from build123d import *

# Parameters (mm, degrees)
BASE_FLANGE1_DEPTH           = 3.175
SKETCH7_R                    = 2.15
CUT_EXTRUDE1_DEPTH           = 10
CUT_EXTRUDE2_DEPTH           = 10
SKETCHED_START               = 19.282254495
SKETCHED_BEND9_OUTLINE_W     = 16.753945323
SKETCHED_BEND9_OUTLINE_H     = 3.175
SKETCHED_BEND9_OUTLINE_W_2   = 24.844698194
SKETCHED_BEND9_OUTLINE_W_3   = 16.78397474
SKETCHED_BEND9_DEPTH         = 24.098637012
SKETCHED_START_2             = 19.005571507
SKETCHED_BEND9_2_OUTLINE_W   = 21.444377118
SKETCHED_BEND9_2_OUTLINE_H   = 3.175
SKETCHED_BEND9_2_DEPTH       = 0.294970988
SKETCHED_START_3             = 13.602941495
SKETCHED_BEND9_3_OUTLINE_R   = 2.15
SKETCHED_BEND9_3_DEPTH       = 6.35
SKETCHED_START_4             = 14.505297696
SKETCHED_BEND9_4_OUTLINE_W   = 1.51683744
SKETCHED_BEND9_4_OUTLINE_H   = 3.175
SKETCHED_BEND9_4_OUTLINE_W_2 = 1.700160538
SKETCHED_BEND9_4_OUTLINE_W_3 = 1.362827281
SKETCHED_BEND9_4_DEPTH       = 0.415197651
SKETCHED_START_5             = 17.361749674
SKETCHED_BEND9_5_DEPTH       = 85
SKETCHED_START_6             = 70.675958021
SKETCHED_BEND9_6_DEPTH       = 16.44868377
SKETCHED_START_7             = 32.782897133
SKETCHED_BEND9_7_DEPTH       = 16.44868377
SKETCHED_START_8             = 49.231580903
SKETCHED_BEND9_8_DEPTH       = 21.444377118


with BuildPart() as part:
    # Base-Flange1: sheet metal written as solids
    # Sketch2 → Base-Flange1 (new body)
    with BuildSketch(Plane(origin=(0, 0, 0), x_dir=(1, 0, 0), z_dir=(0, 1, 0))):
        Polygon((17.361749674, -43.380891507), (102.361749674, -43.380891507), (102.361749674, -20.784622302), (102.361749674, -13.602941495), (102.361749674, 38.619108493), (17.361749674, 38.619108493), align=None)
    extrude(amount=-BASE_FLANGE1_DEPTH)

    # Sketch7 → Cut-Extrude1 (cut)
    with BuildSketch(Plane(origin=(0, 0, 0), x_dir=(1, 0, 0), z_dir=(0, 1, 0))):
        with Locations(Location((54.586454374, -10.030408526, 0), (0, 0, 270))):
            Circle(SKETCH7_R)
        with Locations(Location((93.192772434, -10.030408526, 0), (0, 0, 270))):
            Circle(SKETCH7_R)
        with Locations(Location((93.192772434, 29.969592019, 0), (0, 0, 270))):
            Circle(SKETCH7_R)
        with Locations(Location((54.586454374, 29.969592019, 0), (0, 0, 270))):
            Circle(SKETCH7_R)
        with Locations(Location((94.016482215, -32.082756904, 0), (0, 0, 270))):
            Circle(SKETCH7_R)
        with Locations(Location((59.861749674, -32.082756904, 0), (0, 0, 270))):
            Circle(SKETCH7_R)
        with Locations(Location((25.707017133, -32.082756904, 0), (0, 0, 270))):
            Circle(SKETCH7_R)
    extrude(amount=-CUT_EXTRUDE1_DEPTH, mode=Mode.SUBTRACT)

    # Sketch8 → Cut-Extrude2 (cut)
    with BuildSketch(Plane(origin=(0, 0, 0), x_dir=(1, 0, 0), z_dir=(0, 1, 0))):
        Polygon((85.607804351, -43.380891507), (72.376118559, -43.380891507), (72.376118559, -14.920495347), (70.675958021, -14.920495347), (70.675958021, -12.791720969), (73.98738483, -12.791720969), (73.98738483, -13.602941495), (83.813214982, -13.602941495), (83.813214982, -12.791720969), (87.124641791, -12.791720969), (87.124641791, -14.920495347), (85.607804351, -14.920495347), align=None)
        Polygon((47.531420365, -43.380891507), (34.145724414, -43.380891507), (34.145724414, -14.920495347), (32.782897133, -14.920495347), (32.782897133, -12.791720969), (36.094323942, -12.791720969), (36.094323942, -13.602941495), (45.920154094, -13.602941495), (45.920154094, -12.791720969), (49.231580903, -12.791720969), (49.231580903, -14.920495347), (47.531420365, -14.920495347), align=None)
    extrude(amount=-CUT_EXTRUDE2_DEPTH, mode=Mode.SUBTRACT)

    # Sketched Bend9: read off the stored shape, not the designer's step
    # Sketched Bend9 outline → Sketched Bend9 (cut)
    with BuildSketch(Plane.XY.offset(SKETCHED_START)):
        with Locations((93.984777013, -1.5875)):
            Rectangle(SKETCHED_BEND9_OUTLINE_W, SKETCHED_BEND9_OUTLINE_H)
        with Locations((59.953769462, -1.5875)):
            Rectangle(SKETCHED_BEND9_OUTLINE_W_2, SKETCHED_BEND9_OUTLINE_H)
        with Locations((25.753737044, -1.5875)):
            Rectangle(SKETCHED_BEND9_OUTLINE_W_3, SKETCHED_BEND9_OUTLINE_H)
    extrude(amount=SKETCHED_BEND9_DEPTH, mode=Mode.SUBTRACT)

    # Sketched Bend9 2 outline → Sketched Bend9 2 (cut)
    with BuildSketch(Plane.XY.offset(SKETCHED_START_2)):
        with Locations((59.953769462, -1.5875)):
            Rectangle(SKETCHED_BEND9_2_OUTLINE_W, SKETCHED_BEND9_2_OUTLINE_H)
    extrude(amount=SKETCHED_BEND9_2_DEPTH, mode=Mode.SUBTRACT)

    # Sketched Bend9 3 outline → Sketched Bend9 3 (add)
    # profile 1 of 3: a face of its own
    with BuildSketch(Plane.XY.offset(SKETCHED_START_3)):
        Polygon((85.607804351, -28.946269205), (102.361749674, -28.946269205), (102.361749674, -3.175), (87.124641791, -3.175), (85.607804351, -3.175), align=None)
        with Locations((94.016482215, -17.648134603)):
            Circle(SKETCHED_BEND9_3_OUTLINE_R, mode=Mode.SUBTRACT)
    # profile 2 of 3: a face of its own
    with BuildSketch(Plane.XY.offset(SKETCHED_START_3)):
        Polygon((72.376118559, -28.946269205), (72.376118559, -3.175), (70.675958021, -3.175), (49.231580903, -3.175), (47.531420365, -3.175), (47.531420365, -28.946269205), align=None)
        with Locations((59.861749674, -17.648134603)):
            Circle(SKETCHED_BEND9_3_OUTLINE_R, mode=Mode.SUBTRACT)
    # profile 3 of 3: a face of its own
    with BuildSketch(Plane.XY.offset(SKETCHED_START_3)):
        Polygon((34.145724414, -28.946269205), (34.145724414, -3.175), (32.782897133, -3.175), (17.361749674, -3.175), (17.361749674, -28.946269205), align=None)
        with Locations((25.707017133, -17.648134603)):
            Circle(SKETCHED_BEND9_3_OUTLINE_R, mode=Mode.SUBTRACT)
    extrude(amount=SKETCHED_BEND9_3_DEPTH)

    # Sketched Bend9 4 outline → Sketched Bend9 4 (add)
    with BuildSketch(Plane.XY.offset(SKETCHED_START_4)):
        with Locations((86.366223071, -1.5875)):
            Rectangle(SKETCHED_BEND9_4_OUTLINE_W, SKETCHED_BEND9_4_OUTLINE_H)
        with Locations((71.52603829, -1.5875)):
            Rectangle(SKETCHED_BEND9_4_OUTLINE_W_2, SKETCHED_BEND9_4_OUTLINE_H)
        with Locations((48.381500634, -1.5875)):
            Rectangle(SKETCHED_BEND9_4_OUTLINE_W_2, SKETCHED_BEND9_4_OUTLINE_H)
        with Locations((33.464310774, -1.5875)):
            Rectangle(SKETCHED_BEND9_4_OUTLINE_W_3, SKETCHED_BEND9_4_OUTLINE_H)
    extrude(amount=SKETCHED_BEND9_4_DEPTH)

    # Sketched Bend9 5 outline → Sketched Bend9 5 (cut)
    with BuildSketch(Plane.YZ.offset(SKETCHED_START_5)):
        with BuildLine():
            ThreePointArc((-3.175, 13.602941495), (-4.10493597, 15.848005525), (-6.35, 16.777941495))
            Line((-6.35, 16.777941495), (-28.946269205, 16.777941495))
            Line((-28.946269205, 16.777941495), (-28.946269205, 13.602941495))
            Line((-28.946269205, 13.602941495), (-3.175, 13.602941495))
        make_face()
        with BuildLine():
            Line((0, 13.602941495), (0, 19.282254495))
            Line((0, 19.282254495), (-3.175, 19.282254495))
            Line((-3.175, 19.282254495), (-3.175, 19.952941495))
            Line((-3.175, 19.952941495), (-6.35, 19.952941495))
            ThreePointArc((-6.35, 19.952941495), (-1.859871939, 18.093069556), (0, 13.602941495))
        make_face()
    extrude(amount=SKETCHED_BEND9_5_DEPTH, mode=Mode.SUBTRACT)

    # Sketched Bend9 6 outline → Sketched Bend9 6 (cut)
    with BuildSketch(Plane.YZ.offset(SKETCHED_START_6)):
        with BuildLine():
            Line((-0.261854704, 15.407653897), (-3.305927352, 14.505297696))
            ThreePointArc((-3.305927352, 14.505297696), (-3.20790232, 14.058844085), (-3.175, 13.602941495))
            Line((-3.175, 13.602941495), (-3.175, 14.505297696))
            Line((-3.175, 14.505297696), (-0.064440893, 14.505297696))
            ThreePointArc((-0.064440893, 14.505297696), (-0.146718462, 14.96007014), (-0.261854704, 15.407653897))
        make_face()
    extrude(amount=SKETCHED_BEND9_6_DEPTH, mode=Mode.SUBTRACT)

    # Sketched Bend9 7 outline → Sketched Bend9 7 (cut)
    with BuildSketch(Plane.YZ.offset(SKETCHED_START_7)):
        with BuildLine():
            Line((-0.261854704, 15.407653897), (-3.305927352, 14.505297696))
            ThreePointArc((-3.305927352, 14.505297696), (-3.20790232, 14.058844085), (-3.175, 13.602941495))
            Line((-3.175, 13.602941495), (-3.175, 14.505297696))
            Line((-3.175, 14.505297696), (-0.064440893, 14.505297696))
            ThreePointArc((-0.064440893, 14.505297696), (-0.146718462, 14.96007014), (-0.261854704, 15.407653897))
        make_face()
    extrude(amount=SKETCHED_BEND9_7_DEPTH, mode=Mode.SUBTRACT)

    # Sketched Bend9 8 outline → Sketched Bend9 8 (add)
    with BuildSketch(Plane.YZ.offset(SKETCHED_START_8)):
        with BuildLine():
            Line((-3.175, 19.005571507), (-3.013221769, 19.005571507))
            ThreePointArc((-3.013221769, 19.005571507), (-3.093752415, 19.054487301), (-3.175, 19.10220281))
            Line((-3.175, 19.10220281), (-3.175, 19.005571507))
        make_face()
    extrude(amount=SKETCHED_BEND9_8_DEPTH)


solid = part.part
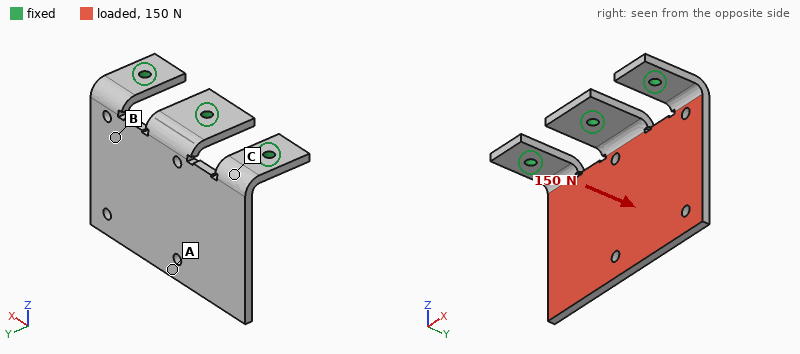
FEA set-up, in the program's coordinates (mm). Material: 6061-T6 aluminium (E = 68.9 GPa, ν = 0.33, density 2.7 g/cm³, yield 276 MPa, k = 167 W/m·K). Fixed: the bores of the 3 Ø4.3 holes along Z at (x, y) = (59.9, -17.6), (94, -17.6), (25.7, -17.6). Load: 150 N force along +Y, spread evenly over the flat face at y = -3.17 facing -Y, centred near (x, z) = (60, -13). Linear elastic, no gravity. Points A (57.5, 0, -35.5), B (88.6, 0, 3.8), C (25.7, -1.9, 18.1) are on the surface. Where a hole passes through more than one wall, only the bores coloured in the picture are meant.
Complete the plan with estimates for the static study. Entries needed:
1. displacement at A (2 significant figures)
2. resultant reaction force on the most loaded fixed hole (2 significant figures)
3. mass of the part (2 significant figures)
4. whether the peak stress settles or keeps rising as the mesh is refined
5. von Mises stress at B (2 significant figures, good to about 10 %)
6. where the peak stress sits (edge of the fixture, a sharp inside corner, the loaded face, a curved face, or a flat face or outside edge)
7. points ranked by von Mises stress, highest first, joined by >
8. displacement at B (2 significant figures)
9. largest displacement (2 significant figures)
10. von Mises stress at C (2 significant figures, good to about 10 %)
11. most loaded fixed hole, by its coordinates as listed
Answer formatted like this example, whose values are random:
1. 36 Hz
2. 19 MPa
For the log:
1. 0.61 mm
2. 81 N
3. 52 g
4. keeps rising
5. 16 MPa
6. edge of the fixture
7. C > B > A
8. 0.14 mm
9. 0.65 mm
10. 34 MPa
11. (59.9, -17.6)
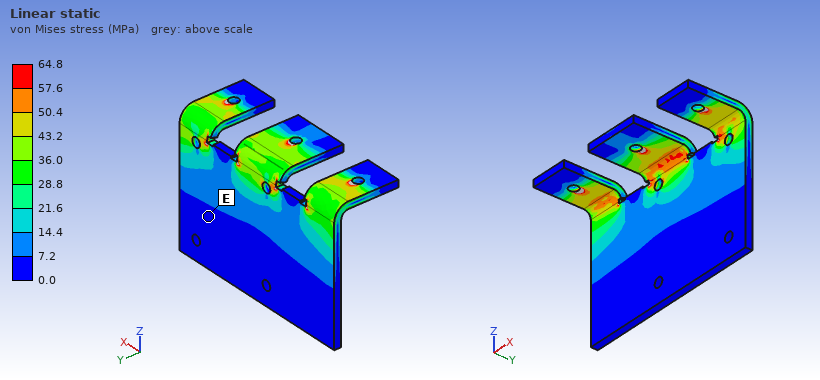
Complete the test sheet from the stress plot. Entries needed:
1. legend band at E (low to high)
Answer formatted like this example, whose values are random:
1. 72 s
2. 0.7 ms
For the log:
1. 0.0 to 7.2 MPa
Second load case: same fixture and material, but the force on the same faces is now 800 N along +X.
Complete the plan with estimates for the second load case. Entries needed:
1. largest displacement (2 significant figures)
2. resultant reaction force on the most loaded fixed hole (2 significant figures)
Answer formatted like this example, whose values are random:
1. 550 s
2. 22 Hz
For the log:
1. 0.31 mm
2. 410 N
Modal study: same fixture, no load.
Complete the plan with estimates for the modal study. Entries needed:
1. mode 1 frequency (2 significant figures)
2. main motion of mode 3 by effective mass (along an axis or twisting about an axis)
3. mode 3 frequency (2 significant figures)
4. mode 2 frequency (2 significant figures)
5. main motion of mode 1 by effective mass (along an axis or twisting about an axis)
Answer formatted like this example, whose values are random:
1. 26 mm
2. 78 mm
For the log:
1. 490 Hz
2. along X
3. 2100 Hz
4. 1100 Hz
5. along Y
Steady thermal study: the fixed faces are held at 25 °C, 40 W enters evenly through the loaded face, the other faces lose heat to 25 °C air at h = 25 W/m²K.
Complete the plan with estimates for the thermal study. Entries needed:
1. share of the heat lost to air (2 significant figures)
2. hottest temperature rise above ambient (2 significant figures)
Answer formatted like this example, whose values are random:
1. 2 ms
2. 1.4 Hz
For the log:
1. 15 %
2. 46 K
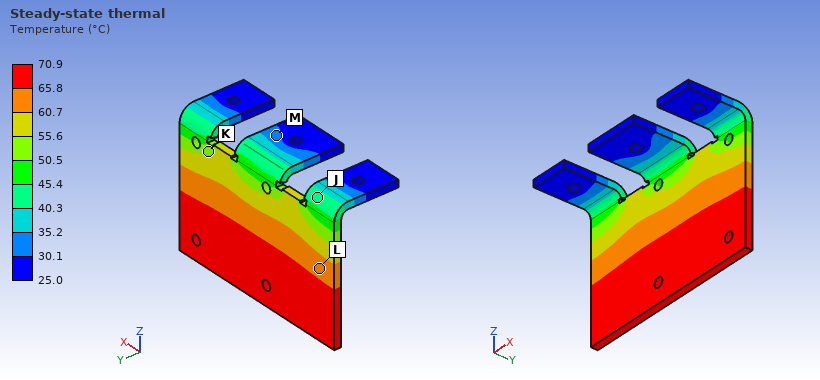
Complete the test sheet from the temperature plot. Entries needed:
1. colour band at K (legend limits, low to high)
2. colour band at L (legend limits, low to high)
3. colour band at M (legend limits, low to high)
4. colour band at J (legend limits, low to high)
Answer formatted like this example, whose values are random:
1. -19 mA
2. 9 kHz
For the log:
1. 50.5 to 55.6 °C
2. 60.7 to 65.8 °C
3. 30.1 to 35.2 °C
4. 40.3 to 45.4 °C
